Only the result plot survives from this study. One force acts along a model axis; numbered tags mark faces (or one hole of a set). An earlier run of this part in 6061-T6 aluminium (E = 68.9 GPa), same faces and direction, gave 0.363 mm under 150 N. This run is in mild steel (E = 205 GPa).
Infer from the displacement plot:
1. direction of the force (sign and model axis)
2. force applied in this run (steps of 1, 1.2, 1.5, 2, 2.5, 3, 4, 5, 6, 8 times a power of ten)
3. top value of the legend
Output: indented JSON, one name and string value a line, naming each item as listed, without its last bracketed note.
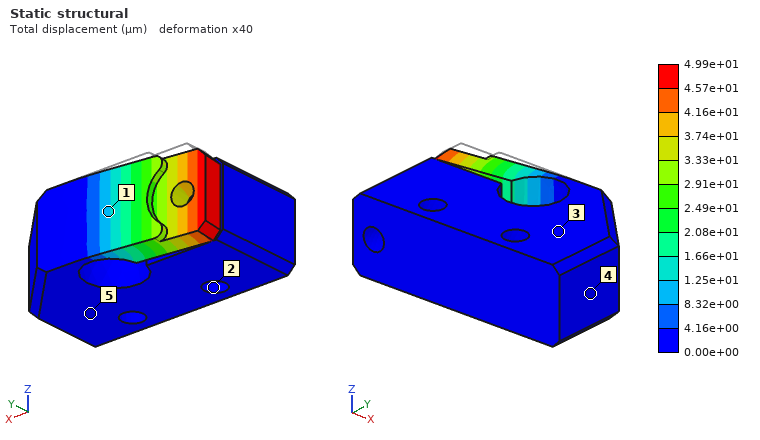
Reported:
{
  "direction of the force": "-Y",
  "force applied in this run": "60 N",
  "top value of the legend": "4.99e+01 µm"
}
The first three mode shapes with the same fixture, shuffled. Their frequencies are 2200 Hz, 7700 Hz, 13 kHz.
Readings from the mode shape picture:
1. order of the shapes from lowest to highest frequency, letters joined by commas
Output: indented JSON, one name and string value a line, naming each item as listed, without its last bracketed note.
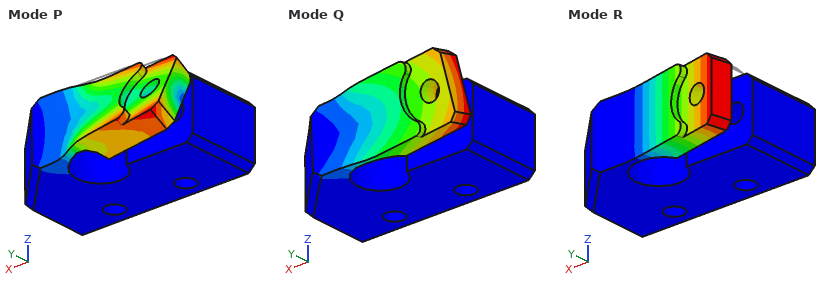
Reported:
{
  "order of the shapes from lowest to highest frequency, letters joined by commas": "R, Q, P"
}
